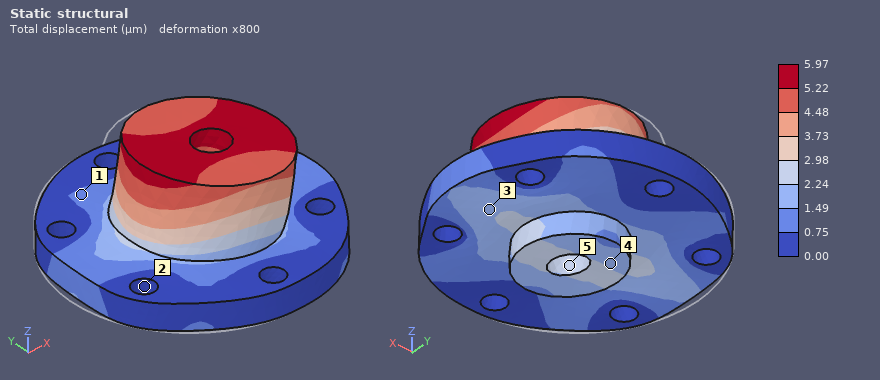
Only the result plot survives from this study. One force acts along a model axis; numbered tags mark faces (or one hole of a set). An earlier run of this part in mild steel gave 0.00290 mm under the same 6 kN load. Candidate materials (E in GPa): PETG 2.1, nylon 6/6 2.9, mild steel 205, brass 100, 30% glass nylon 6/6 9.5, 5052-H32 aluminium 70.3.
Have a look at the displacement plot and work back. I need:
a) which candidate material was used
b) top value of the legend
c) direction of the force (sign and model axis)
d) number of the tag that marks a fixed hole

brass
5.97 µm
+X
2
